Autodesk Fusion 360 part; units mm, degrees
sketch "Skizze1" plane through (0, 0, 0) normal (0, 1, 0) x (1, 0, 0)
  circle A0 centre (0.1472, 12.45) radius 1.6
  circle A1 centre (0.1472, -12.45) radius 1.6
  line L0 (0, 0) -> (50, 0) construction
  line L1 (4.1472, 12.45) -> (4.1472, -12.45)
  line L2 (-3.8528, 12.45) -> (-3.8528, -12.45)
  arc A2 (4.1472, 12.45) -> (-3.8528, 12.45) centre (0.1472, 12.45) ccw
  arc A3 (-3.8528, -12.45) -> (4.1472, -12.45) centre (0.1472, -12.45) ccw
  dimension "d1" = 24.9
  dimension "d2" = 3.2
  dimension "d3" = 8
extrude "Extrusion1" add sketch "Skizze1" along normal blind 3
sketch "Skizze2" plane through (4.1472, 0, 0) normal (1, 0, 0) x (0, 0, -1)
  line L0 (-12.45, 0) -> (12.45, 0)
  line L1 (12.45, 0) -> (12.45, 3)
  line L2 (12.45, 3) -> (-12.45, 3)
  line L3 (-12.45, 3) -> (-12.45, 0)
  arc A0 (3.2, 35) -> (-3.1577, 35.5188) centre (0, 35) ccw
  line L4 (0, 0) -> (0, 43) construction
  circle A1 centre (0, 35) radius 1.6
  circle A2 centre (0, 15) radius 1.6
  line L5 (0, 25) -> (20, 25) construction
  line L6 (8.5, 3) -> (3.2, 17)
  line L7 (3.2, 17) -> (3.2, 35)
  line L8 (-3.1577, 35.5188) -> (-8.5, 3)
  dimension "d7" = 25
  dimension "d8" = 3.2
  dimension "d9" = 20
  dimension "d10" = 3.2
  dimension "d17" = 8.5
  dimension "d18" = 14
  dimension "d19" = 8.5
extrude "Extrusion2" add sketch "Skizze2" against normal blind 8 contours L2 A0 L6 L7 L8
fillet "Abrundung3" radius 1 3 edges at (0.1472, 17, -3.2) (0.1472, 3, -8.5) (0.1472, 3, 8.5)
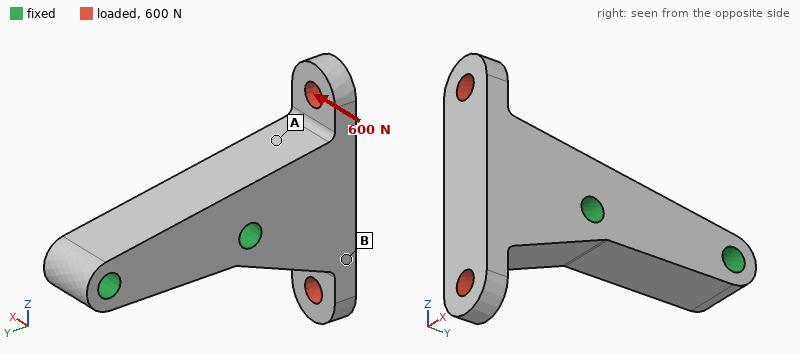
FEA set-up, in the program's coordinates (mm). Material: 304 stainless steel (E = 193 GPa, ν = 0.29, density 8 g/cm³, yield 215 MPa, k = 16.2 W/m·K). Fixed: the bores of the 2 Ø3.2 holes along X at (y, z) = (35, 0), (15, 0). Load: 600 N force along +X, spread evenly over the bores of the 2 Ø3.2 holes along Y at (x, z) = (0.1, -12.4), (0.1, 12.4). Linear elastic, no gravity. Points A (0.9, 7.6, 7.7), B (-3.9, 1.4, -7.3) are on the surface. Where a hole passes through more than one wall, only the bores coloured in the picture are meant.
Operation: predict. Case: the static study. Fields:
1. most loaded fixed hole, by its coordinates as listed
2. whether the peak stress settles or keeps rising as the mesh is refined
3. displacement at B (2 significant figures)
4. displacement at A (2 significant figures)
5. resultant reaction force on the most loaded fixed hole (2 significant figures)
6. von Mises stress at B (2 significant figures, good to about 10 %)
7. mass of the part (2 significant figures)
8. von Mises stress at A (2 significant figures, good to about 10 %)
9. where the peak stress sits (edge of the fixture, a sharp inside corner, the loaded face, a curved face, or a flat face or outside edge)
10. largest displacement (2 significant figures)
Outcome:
(15, 0)
keeps rising
7.8 µm
2.9 µm
650 N
43 MPa
27 g
23 MPa
edge of the fixture
14 µm
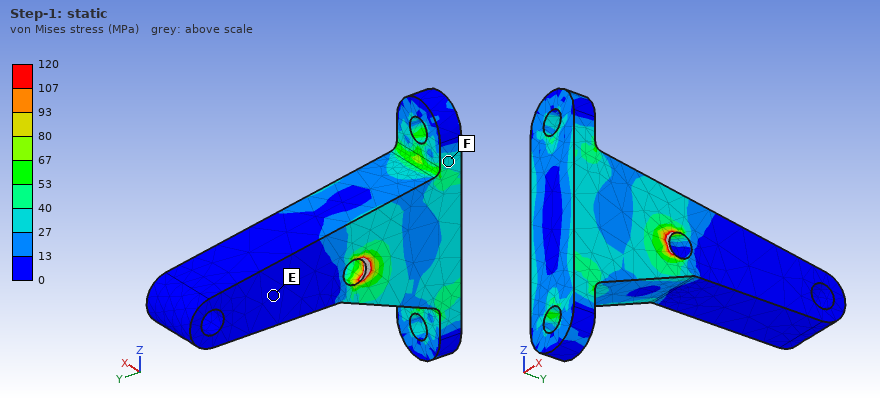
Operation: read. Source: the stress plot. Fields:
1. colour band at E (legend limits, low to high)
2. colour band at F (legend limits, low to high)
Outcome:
0 to 13 MPa
27 to 40 MPa
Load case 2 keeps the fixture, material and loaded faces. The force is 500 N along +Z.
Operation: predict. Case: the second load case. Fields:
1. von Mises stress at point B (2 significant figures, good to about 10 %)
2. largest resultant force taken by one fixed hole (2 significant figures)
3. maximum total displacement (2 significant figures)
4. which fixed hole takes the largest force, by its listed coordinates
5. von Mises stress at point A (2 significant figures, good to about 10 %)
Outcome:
11 MPa
670 N
10 µm
(15, 0)
12 MPa
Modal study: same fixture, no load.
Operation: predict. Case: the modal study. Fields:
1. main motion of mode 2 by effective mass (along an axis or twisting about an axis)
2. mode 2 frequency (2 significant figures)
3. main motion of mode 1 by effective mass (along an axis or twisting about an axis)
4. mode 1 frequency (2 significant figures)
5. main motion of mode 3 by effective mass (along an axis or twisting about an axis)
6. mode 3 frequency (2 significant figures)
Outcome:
along X
16 kHz
along Z
14 kHz
twisting about Y
18 kHz
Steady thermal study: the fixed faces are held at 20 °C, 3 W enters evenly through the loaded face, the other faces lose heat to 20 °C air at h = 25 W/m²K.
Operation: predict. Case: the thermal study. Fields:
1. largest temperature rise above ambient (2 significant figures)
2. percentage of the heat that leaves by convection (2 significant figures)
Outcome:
47 K
19 %
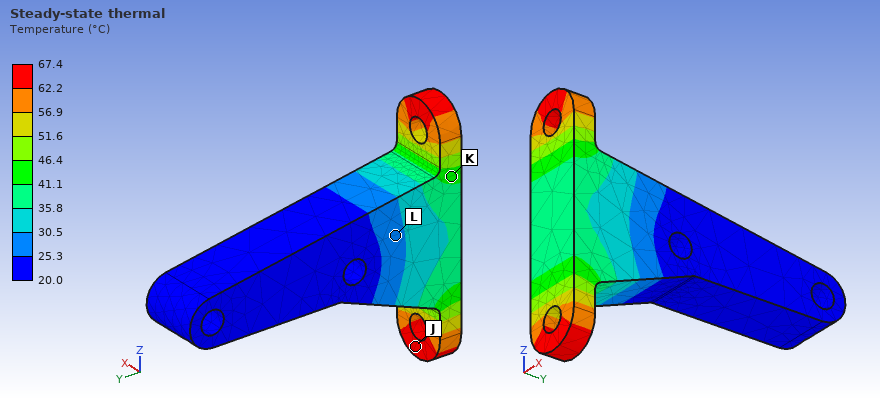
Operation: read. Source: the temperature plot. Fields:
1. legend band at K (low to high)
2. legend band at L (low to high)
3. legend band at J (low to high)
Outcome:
41.1 to 46.4 °C
25.3 to 30.5 °C
62.2 to 67.4 °C
